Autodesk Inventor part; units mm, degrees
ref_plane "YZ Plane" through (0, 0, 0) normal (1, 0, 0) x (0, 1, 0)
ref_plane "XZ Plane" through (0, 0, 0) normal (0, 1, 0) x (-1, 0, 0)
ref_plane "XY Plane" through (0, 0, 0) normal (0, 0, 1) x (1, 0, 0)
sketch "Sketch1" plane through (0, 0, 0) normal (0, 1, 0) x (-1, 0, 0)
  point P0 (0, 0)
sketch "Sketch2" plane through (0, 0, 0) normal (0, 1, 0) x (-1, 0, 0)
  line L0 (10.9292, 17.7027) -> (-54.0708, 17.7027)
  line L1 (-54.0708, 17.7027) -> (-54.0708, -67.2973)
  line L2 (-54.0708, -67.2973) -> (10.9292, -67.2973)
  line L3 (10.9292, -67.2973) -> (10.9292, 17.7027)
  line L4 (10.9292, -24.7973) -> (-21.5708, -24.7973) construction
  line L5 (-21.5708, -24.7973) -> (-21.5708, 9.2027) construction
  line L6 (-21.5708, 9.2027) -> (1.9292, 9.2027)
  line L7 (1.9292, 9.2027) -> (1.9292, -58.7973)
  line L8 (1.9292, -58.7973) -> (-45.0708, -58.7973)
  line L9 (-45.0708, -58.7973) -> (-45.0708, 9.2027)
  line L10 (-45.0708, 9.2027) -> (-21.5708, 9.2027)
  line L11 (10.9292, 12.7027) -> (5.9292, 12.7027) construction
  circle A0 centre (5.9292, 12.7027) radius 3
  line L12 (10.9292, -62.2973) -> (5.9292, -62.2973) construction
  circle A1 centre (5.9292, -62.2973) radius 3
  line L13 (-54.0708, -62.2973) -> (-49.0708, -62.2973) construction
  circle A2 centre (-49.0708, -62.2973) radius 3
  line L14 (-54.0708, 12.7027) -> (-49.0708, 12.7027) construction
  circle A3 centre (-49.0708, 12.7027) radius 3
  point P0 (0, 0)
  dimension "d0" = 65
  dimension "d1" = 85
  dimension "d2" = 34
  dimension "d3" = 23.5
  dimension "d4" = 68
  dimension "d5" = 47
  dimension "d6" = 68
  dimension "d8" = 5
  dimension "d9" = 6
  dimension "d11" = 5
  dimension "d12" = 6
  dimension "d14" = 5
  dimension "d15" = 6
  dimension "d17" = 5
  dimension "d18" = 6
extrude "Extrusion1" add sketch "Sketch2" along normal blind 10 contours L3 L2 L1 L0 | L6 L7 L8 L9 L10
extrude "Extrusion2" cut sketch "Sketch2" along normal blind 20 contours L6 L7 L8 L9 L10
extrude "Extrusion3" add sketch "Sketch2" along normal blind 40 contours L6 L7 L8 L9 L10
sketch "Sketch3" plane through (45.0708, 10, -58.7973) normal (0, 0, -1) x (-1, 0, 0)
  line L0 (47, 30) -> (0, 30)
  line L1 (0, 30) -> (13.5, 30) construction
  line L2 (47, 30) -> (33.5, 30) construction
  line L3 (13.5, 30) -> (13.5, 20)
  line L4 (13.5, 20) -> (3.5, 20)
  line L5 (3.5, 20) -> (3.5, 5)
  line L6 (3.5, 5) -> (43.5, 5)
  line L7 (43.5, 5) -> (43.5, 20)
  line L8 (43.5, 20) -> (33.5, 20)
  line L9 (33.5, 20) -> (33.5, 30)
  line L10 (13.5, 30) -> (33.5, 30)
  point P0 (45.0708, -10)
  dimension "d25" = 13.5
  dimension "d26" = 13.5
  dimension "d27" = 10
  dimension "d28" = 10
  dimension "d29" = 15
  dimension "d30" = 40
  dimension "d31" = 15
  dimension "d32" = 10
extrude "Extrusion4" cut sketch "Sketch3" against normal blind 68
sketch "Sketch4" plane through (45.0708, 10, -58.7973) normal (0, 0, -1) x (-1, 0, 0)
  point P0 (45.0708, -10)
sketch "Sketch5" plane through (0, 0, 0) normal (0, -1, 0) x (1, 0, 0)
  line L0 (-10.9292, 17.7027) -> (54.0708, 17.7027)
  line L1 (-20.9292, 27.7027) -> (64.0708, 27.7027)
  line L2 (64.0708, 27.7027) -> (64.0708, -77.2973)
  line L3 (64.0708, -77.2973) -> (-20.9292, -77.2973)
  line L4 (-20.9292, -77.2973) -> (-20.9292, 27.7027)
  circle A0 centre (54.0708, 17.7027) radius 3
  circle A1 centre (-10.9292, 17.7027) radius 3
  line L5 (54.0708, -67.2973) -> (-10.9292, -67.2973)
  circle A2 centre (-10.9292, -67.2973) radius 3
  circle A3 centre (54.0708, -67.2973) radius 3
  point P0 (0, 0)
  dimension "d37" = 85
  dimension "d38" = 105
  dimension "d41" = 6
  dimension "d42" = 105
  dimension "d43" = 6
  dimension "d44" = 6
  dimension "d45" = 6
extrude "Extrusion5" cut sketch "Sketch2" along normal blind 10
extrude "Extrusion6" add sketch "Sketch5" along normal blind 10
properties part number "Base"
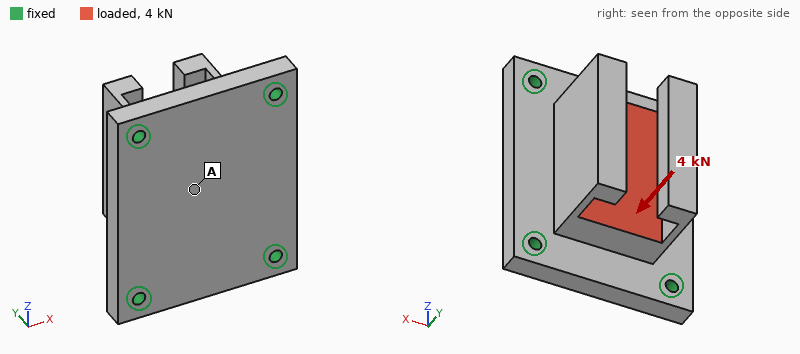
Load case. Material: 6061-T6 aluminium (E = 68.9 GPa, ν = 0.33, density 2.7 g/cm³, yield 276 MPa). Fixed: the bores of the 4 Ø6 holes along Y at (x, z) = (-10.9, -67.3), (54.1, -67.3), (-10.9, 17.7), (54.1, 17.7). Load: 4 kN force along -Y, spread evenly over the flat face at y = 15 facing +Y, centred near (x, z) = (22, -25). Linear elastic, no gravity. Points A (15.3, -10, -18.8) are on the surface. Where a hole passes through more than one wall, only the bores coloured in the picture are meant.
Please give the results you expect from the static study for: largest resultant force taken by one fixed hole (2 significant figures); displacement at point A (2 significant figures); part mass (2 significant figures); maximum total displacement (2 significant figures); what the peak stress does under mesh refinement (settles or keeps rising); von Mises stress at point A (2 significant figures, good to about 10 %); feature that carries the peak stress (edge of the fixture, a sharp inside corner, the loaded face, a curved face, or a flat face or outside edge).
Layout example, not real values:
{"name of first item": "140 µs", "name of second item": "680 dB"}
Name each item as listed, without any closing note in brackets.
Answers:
{"largest resultant force taken by one fixed hole": "1.1 kN", "displacement at point A": "11 µm", "part mass": "440 g", "maximum total displacement": "11 µm", "what the peak stress does under mesh refinement": "keeps rising", "von Mises stress at point A": "3.4 MPa", "feature that carries the peak stress": "edge of the fixture"}
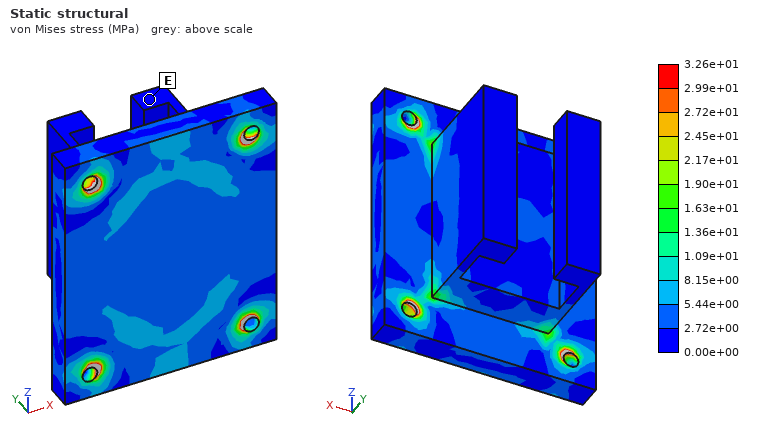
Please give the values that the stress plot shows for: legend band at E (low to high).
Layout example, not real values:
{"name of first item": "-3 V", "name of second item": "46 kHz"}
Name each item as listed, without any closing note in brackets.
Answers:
{"legend band at E": "0.00e+00 to 2.72e+00 MPa"}
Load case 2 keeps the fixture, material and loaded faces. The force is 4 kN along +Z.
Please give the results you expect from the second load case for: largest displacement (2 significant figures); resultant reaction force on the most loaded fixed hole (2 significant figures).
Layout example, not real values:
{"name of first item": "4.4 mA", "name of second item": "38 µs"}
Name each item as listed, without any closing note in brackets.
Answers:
{"largest displacement": "7.9 µm", "resultant reaction force on the most loaded fixed hole": "1.2 kN"}
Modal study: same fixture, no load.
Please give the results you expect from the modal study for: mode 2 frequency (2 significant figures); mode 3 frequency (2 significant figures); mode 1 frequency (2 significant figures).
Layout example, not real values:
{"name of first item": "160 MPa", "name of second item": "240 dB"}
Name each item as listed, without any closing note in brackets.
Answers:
{"mode 2 frequency": "2100 Hz", "mode 3 frequency": "4600 Hz", "mode 1 frequency": "2100 Hz"}
